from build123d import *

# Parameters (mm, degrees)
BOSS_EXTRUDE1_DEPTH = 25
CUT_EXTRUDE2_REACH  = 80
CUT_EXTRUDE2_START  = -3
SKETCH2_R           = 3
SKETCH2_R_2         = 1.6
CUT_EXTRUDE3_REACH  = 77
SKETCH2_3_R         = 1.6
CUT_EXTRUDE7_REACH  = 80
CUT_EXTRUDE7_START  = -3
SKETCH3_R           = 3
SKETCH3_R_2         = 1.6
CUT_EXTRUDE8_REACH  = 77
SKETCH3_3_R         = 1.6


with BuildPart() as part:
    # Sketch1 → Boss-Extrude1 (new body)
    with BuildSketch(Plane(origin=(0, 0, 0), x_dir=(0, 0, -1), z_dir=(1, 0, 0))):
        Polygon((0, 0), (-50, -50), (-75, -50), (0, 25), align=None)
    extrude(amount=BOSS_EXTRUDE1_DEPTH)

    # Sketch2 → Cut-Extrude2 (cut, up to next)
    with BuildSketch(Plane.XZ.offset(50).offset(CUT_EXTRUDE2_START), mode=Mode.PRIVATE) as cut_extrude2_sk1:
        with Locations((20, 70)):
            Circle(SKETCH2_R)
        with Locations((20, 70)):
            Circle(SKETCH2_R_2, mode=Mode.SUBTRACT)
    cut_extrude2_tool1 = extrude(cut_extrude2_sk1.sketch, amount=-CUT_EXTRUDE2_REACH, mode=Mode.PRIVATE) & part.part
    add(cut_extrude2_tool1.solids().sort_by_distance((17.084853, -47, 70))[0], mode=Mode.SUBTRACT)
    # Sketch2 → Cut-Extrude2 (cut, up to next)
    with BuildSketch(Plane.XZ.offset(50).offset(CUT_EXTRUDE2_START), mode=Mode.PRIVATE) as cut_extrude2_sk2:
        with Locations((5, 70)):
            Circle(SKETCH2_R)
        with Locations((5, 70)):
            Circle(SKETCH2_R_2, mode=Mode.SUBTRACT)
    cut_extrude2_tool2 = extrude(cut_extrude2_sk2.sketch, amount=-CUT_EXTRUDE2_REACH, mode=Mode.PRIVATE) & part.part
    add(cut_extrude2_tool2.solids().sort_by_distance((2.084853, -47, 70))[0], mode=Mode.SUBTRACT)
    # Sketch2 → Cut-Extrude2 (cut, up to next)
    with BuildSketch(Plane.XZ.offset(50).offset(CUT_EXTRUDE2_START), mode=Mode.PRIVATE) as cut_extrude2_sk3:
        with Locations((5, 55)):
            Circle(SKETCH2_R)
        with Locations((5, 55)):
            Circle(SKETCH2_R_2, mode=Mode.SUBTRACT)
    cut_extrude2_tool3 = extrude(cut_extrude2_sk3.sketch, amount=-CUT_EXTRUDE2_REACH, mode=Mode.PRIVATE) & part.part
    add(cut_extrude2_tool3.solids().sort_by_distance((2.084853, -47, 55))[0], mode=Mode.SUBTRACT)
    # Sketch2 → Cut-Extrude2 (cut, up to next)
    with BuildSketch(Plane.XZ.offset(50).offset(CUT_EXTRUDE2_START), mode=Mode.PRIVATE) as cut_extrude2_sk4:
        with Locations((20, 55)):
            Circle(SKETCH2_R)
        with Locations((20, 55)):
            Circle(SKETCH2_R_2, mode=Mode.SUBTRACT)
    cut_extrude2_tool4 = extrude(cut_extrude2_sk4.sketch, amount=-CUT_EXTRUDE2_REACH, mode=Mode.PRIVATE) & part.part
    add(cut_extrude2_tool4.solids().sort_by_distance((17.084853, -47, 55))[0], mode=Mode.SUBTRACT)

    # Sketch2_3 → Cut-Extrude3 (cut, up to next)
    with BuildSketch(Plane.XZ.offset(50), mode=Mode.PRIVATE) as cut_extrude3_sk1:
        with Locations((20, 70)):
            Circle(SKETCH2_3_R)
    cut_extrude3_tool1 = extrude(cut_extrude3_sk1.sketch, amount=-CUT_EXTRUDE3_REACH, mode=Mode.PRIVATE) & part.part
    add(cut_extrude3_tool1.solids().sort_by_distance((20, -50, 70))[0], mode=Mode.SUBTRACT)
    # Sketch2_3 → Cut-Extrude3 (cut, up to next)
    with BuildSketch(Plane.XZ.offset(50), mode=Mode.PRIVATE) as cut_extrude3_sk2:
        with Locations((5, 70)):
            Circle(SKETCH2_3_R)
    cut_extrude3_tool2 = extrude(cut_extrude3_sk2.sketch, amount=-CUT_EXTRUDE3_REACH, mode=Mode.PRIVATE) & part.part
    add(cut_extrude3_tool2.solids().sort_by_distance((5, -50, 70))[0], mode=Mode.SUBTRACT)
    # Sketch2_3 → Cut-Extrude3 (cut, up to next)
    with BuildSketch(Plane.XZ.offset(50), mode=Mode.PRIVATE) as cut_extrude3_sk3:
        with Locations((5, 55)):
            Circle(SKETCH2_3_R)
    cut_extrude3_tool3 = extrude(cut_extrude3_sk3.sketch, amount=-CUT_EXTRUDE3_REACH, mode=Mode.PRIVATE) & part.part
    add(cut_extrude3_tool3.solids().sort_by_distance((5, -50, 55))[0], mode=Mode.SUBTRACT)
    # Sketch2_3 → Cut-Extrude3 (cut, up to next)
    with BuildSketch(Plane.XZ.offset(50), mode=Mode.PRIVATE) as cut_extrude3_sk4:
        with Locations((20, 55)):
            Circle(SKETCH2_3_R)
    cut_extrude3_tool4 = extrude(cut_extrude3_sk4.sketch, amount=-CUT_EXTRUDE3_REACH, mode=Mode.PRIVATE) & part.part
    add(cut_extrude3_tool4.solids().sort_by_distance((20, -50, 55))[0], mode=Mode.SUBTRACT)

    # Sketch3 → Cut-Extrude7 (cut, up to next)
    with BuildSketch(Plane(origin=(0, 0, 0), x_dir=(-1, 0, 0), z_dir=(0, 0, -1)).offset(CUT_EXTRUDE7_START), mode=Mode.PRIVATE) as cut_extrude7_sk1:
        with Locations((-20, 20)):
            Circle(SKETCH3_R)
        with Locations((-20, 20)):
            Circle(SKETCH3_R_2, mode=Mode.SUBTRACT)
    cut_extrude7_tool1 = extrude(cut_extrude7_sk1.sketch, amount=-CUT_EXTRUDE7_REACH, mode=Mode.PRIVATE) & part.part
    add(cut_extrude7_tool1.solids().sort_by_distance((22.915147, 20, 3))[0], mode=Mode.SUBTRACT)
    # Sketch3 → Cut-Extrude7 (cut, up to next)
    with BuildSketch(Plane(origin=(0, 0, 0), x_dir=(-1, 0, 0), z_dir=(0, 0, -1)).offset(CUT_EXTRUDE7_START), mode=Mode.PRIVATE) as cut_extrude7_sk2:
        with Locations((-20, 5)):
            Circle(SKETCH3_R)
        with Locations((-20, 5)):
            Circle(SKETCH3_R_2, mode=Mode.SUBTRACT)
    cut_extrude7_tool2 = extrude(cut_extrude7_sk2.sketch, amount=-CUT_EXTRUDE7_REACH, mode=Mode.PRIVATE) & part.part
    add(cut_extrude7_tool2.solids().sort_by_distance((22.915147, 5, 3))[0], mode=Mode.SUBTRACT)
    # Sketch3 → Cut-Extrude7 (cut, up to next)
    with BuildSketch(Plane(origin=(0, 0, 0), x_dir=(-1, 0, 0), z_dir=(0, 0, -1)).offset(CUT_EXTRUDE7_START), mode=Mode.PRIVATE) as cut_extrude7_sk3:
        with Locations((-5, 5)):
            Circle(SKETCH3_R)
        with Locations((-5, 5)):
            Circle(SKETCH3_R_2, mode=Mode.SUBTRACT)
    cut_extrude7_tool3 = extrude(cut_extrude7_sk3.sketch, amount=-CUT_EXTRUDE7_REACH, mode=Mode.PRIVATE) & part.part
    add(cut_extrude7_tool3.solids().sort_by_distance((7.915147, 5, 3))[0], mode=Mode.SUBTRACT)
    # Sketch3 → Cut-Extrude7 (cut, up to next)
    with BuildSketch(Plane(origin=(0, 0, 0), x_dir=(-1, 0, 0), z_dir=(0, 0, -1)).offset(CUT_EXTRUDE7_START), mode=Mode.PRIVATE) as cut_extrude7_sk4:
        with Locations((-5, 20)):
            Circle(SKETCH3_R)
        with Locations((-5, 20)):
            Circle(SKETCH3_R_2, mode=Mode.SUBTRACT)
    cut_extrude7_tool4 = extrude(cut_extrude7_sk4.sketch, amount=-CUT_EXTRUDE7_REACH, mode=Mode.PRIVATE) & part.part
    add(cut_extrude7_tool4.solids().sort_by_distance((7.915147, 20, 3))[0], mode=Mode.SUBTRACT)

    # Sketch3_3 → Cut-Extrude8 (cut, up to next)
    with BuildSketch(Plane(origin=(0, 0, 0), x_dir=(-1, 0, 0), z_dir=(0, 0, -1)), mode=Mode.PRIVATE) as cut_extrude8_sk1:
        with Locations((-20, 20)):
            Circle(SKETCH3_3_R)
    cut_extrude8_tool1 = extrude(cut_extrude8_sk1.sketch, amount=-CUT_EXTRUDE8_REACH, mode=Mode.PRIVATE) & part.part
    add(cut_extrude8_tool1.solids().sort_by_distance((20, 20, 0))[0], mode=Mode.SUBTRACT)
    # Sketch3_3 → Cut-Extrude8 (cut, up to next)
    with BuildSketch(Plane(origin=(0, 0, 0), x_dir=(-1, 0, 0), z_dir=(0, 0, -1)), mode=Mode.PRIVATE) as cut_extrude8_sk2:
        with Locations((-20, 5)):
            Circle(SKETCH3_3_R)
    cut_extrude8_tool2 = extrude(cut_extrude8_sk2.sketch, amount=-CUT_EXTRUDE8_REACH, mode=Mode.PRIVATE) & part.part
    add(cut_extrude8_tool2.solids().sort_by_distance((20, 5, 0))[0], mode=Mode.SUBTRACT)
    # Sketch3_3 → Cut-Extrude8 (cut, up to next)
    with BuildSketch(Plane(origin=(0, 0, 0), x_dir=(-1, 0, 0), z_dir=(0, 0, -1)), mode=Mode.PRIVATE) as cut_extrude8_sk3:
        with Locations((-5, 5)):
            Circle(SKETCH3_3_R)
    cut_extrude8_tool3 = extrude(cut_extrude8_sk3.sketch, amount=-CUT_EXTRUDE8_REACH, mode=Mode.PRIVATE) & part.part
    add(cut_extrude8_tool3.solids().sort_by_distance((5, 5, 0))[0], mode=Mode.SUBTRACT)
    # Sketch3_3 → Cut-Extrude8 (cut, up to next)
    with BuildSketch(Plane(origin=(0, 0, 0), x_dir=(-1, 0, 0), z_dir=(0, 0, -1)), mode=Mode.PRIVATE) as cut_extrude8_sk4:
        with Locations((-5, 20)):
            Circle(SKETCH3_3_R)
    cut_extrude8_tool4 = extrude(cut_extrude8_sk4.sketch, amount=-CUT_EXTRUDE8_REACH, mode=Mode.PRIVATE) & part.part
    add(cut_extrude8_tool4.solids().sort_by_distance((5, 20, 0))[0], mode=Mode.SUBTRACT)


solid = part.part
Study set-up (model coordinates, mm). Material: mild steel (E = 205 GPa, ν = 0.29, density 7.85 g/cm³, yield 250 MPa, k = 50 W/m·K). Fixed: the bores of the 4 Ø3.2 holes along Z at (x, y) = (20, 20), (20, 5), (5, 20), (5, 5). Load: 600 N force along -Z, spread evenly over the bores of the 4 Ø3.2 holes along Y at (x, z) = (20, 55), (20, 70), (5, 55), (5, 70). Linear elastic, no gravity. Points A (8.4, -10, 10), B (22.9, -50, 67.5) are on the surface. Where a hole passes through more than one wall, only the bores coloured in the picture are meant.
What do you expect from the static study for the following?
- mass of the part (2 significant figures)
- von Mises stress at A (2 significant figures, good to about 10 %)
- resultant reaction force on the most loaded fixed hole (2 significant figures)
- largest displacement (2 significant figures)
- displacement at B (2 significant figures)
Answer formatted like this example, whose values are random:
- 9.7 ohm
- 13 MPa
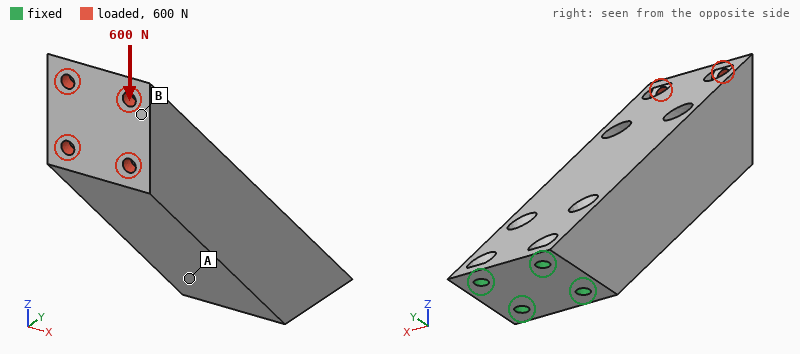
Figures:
- 290 g
- 22 MPa
- 1.4 kN
- 69 µm
- 64 µm
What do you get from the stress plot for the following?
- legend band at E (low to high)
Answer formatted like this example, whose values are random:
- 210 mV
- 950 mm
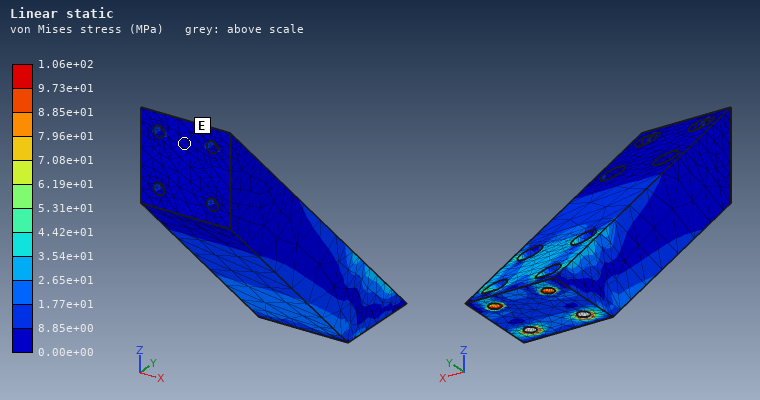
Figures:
- 0.00e+00 to 8.85e+00 MPa
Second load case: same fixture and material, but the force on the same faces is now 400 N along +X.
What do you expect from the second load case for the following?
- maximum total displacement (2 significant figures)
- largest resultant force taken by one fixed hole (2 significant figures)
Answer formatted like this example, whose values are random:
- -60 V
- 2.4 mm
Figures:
- 34 µm
- 1.3 kN
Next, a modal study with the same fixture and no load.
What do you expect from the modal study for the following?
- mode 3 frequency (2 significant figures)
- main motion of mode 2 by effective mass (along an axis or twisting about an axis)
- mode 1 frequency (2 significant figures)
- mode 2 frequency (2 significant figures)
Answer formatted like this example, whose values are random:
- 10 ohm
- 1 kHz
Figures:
- 7600 Hz
- along X
- 1500 Hz
- 2100 Hz
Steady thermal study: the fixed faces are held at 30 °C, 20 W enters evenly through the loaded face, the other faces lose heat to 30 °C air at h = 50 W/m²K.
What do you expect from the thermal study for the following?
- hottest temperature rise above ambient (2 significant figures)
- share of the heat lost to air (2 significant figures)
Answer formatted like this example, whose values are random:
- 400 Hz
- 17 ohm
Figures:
- 65 K
- 58 %
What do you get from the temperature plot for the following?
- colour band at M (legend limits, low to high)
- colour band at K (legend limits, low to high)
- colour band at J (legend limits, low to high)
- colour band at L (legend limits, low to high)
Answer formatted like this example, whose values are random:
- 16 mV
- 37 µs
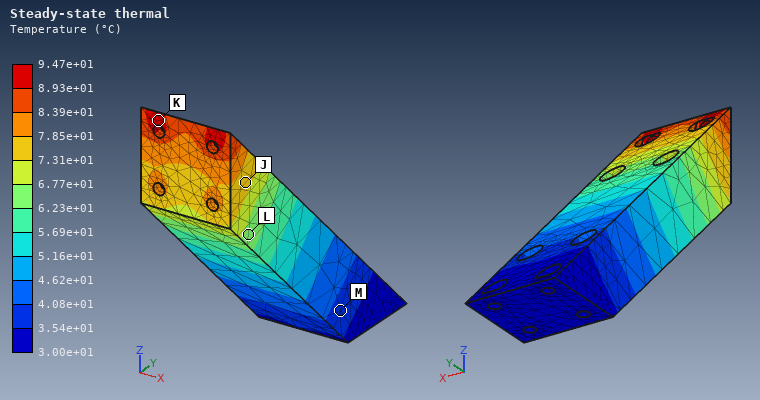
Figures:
- 3.54e+01 to 4.08e+01 °C
- 8.93e+01 to 9.47e+01 °C
- 7.31e+01 to 7.85e+01 °C
- 6.23e+01 to 6.77e+01 °C
